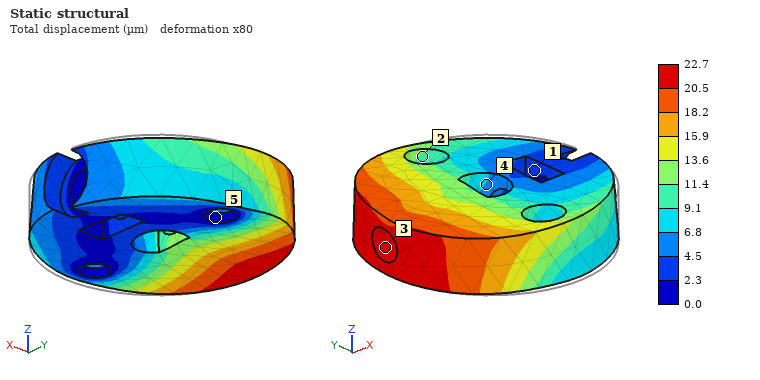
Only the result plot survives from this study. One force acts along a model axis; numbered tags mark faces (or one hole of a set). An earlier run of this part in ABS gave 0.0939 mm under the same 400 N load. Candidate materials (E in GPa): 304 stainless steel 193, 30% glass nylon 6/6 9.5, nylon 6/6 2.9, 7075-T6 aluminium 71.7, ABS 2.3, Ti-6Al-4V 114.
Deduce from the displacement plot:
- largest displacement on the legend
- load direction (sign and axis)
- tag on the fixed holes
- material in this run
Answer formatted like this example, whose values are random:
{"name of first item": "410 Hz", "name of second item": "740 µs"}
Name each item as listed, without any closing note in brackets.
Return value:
{"largest displacement on the legend": "22.7 µm", "load direction": "+Y", "tag on the fixed holes": "5", "material in this run": "30% glass nylon 6/6"}
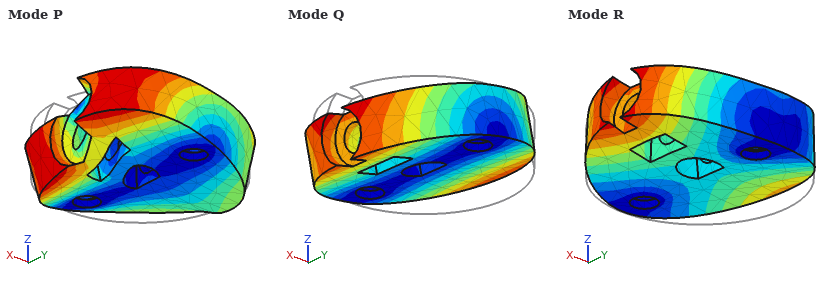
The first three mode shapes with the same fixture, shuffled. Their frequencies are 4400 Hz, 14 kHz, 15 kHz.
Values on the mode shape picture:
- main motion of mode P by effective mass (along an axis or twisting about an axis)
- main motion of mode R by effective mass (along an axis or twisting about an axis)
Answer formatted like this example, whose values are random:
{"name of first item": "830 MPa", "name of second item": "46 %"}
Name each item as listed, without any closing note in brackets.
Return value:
{"main motion of mode P by effective mass": "twisting about Z", "main motion of mode R by effective mass": "along Z"}
